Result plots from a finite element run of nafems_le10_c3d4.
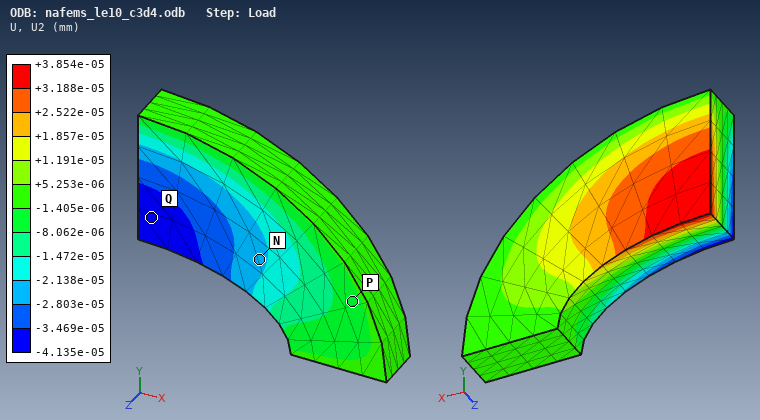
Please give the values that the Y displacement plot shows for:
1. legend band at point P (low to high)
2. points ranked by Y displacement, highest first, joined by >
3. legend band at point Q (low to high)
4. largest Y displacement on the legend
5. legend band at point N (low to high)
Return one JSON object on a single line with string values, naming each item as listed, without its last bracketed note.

{"legend band at point P": "-8.062e-06 to -1.405e-06 mm", "points ranked by Y displacement, highest first, joined by >": "P > N > Q", "legend band at point Q": "-4.135e-05 to -3.469e-05 mm", "largest Y displacement on the legend": "+3.854e-05 mm", "legend band at point N": "-2.803e-05 to -2.138e-05 mm"}
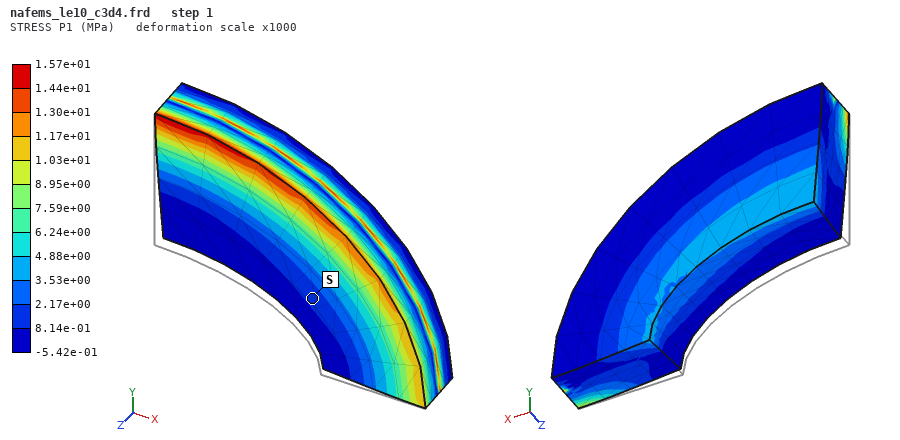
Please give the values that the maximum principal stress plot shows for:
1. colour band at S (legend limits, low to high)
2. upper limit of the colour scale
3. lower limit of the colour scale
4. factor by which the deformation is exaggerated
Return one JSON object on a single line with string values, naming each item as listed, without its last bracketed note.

{"colour band at S": "8.14e-01 to 2.17e+00 MPa", "upper limit of the colour scale": "1.57e+01 MPa", "lower limit of the colour scale": "-5.42e-01 MPa", "factor by which the deformation is exaggerated": "1000"}
